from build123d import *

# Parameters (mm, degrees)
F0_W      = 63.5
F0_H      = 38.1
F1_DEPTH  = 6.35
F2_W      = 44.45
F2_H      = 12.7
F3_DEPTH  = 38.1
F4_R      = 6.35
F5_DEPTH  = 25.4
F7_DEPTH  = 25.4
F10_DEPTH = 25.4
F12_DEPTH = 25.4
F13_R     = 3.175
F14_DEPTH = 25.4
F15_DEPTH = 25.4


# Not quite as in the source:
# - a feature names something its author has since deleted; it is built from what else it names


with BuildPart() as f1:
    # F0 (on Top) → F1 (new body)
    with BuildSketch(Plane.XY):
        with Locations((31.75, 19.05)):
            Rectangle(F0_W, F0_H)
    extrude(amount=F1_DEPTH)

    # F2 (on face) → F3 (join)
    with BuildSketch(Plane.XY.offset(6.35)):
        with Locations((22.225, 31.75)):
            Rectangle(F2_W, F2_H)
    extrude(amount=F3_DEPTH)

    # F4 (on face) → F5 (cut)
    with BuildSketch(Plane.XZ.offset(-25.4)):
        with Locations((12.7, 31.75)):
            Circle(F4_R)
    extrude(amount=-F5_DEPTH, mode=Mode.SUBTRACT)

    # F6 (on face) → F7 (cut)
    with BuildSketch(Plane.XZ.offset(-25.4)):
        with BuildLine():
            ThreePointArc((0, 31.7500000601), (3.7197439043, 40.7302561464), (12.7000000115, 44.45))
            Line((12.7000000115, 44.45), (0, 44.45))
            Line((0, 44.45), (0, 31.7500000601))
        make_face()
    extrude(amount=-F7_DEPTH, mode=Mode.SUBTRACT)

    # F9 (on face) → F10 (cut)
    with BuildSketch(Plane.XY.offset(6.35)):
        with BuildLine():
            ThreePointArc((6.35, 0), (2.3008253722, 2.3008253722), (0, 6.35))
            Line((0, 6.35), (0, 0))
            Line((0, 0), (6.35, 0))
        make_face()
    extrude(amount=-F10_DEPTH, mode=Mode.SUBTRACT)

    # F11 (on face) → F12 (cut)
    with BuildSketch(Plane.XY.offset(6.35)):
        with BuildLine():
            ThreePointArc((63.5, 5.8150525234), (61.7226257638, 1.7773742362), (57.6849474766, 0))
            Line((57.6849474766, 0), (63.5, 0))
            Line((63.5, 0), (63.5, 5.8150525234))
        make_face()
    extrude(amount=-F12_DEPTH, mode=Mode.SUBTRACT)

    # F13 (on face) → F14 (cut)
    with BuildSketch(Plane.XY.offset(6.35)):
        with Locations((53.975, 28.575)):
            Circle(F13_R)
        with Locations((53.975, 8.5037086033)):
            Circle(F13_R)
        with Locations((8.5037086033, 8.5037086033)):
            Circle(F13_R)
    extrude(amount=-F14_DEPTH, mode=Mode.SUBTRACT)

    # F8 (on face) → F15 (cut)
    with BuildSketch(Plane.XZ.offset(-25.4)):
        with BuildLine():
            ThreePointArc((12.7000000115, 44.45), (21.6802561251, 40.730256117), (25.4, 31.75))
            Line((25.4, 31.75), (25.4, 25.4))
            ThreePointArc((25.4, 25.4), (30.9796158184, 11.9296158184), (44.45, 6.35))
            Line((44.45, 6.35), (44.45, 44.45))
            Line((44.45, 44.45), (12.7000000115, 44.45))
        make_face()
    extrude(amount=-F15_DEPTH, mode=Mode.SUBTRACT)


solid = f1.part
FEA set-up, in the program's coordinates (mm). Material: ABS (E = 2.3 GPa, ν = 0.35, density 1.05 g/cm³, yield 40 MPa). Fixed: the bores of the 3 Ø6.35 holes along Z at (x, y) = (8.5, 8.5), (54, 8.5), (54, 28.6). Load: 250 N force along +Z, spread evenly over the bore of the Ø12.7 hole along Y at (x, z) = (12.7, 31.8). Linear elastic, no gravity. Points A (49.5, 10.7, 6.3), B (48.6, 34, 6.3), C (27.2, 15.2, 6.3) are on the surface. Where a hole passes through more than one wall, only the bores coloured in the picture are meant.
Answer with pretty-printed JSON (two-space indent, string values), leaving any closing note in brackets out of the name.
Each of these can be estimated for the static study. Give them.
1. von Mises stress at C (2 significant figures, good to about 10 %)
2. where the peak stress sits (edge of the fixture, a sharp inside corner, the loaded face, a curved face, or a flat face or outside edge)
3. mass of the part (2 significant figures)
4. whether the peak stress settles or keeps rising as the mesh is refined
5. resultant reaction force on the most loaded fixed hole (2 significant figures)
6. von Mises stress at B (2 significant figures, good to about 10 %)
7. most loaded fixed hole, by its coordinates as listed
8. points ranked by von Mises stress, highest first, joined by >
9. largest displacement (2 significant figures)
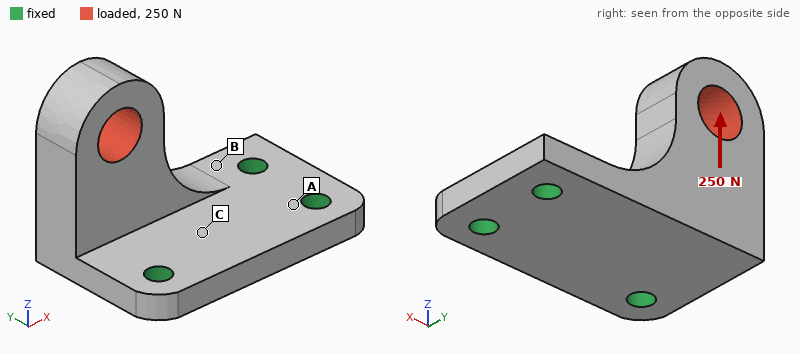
{
  "von Mises stress at C": "4.4 MPa",
  "where the peak stress sits": "edge of the fixture",
  "mass of the part": "27 g",
  "whether the peak stress settles or keeps rising as the mesh is refined": "keeps rising",
  "resultant reaction force on the most loaded fixed hole": "200 N",
  "von Mises stress at B": "7.6 MPa",
  "most loaded fixed hole, by its coordinates as listed": "(8.5, 8.5)",
  "points ranked by von Mises stress, highest first, joined by >": "B > C > A",
  "largest displacement": "0.91 mm"
}
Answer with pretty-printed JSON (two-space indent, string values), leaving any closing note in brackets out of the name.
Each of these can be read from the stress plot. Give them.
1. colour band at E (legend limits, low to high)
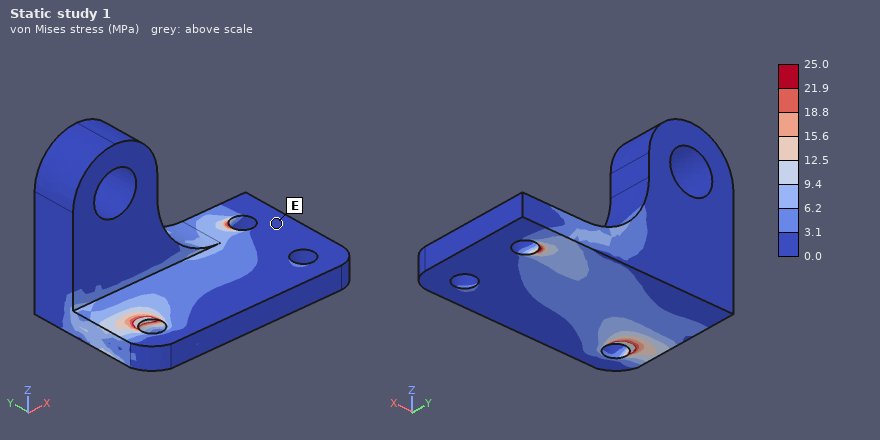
{
  "colour band at E": "0.0 to 3.1 MPa"
}
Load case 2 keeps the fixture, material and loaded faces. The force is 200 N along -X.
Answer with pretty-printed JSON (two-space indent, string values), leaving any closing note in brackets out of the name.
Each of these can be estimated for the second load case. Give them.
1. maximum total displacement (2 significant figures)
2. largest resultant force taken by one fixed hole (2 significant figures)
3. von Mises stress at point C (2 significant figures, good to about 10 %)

{
  "maximum total displacement": "0.60 mm",
  "largest resultant force taken by one fixed hole": "150 N",
  "von Mises stress at point C": "3.3 MPa"
}
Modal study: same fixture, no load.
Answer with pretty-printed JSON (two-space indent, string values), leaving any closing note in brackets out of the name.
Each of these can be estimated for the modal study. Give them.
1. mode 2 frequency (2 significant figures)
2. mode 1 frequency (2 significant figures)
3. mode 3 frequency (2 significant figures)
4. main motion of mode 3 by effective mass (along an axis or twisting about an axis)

{
  "mode 2 frequency": "1600 Hz",
  "mode 1 frequency": "710 Hz",
  "mode 3 frequency": "2300 Hz",
  "main motion of mode 3 by effective mass": "along Z"
}
